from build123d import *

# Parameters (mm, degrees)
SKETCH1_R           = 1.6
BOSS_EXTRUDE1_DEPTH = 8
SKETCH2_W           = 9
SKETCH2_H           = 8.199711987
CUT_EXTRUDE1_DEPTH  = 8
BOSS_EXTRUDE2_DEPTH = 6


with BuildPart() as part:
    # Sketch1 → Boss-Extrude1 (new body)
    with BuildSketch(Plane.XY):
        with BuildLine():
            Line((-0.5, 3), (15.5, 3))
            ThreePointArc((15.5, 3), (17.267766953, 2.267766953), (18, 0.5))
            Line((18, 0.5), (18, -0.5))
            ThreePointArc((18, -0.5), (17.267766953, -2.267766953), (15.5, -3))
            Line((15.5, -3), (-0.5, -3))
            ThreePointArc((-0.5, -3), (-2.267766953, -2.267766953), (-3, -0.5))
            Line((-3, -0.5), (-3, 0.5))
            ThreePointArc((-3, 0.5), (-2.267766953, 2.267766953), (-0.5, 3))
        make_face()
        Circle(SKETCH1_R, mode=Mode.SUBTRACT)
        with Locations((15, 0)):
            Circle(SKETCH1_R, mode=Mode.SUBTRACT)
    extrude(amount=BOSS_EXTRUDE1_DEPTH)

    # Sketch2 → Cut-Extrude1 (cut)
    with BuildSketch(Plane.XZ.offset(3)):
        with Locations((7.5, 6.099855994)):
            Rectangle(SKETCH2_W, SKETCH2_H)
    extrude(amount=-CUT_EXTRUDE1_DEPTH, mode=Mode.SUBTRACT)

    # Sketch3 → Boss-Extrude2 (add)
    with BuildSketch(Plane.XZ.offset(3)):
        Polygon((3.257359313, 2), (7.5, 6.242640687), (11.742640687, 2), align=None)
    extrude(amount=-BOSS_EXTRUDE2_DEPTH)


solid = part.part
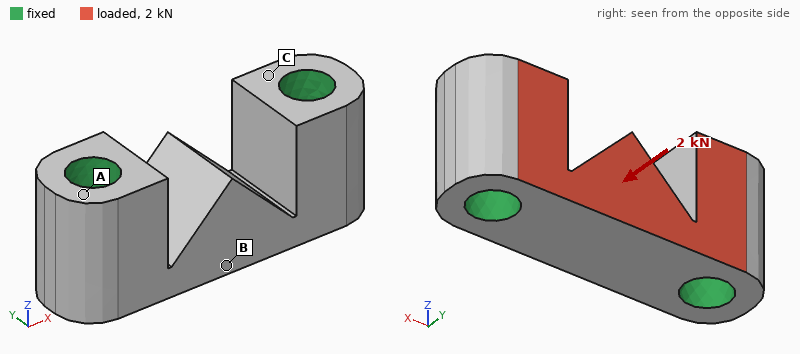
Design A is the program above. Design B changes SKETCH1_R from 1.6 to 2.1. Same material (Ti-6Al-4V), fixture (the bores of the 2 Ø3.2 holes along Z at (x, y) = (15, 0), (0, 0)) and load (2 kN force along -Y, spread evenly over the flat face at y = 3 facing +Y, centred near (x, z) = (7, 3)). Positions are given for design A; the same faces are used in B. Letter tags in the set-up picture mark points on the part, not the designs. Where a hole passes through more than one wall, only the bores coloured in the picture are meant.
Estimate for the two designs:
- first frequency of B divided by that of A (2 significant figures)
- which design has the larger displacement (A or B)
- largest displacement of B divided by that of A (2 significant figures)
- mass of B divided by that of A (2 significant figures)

1.0
A
0.91
0.85
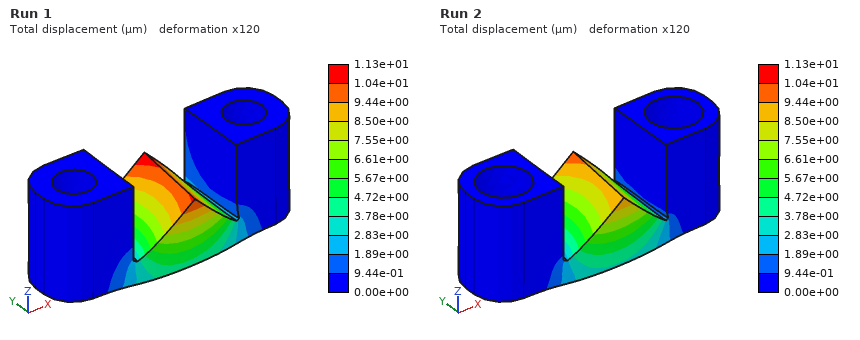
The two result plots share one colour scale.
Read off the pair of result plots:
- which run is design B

Run 2
